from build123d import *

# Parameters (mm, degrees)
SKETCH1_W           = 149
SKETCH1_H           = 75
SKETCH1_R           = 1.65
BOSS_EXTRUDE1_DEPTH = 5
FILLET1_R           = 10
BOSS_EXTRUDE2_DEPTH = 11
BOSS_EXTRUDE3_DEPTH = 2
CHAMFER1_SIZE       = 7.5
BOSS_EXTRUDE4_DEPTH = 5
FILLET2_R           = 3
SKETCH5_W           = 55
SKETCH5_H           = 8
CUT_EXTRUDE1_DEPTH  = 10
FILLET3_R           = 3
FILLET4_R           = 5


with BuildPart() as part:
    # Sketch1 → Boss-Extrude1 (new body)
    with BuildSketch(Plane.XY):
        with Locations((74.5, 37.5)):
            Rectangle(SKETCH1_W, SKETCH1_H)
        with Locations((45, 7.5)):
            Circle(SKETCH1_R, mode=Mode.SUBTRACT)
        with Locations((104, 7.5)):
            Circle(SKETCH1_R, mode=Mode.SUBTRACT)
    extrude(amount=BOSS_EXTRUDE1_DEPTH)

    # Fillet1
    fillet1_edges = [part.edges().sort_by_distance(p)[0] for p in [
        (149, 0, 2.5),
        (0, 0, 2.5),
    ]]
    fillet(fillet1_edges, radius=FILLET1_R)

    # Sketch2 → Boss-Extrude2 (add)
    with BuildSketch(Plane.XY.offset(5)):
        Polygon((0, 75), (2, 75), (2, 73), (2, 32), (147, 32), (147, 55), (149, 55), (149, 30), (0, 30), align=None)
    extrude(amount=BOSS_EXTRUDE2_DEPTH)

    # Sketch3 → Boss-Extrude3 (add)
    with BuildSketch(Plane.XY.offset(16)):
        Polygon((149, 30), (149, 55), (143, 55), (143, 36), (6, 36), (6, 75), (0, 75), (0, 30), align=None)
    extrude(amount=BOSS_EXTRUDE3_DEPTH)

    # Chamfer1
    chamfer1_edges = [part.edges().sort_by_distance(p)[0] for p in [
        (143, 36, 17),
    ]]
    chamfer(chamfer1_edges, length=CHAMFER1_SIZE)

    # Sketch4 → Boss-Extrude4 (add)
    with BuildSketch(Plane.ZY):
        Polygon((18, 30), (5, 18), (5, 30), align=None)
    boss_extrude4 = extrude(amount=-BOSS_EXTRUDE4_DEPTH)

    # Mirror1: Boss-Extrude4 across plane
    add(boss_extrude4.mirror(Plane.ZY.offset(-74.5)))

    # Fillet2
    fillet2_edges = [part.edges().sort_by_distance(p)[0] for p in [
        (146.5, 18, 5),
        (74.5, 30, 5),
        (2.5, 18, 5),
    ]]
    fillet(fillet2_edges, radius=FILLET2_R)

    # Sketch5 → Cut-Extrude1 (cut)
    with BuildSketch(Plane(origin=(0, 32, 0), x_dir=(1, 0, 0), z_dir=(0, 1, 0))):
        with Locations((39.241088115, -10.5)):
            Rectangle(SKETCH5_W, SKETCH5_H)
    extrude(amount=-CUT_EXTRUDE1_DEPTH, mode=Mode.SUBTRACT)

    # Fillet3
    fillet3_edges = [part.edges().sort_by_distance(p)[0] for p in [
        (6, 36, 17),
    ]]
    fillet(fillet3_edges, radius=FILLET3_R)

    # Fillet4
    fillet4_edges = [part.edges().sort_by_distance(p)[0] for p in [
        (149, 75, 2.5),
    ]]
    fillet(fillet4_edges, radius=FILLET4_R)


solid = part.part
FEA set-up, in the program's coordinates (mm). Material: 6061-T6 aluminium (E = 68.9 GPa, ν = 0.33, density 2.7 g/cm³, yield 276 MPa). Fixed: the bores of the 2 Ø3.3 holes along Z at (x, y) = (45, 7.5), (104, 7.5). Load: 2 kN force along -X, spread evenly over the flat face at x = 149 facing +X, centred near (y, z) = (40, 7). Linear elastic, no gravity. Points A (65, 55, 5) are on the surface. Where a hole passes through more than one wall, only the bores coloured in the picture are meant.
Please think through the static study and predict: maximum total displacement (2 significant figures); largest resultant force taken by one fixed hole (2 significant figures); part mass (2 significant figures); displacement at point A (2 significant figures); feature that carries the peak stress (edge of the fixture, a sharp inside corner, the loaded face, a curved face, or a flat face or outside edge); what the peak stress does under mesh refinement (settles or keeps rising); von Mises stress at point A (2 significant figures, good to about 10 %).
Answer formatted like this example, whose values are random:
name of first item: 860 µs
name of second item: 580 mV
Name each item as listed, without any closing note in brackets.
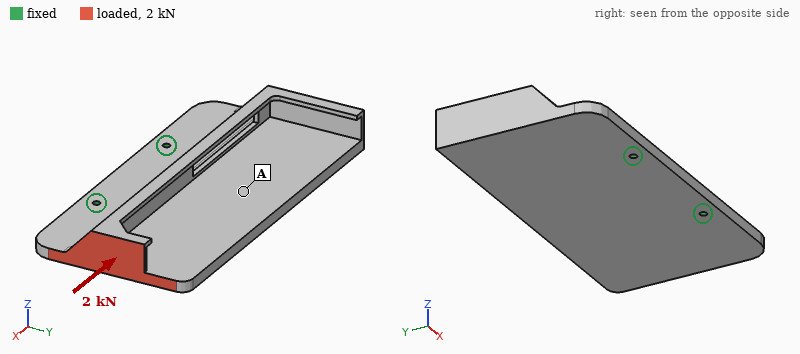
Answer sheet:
maximum total displacement: 0.16 mm
largest resultant force taken by one fixed hole: 1.5 kN
part mass: 170 g
displacement at point A: 0.025 mm
feature that carries the peak stress: edge of the fixture
what the peak stress does under mesh refinement: keeps rising
von Mises stress at point A: 8.4 MPa
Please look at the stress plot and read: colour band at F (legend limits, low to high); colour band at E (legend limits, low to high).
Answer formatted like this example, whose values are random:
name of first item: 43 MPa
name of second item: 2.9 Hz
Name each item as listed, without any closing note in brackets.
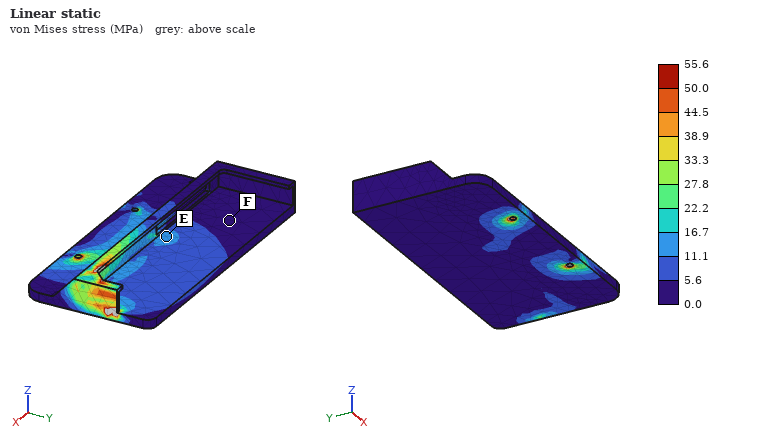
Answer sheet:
colour band at F: 0.0 to 5.6 MPa
colour band at E: 11.1 to 16.7 MPa
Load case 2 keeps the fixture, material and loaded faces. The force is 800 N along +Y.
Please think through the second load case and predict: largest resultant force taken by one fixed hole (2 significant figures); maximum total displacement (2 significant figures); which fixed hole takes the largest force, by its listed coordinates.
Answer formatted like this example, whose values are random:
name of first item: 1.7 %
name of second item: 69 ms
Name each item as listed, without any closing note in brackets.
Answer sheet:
largest resultant force taken by one fixed hole: 1.4 kN
maximum total displacement: 0.19 mm
which fixed hole takes the largest force, by its listed coordinates: (104, 7.5)
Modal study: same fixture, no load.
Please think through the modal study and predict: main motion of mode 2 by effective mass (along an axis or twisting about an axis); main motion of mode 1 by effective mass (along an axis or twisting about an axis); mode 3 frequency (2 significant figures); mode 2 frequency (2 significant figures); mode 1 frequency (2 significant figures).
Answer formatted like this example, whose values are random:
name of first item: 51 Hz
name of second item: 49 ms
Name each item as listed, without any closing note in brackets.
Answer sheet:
main motion of mode 2 by effective mass: twisting about Y
main motion of mode 1 by effective mass: along Z
mode 3 frequency: 1900 Hz
mode 2 frequency: 840 Hz
mode 1 frequency: 620 Hz
